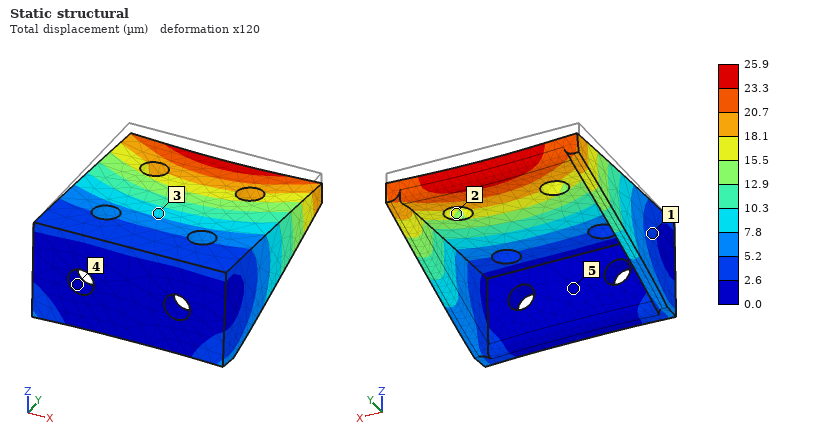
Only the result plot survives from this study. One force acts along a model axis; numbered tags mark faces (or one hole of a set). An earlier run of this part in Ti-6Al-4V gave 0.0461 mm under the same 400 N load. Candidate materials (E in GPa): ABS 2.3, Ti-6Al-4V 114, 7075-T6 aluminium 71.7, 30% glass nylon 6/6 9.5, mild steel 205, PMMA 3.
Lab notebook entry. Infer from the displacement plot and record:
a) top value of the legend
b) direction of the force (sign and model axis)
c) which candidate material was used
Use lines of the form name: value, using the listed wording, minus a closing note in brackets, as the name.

top value of the legend: 25.9 µm
direction of the force: -Z
which candidate material was used: mild steel
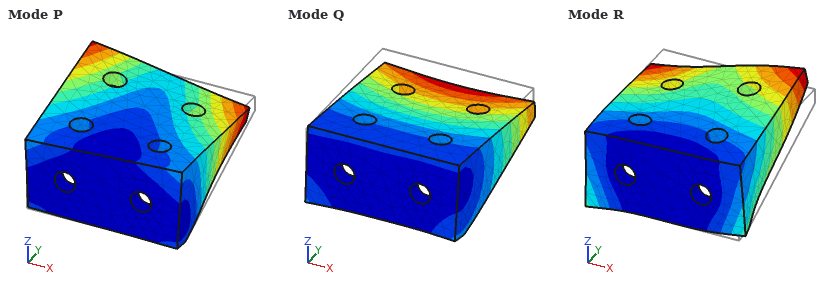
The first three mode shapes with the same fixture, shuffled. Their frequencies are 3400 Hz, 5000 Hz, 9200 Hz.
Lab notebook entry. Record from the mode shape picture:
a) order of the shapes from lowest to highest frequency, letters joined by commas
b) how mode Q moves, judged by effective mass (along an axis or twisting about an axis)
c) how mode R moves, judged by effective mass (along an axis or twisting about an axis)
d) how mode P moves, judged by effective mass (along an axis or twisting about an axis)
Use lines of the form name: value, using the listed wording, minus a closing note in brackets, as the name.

order of the shapes from lowest to highest frequency, letters joined by commas: Q, P, R
how mode Q moves, judged by effective mass: along Z
how mode R moves, judged by effective mass: along X
how mode P moves, judged by effective mass: along X
